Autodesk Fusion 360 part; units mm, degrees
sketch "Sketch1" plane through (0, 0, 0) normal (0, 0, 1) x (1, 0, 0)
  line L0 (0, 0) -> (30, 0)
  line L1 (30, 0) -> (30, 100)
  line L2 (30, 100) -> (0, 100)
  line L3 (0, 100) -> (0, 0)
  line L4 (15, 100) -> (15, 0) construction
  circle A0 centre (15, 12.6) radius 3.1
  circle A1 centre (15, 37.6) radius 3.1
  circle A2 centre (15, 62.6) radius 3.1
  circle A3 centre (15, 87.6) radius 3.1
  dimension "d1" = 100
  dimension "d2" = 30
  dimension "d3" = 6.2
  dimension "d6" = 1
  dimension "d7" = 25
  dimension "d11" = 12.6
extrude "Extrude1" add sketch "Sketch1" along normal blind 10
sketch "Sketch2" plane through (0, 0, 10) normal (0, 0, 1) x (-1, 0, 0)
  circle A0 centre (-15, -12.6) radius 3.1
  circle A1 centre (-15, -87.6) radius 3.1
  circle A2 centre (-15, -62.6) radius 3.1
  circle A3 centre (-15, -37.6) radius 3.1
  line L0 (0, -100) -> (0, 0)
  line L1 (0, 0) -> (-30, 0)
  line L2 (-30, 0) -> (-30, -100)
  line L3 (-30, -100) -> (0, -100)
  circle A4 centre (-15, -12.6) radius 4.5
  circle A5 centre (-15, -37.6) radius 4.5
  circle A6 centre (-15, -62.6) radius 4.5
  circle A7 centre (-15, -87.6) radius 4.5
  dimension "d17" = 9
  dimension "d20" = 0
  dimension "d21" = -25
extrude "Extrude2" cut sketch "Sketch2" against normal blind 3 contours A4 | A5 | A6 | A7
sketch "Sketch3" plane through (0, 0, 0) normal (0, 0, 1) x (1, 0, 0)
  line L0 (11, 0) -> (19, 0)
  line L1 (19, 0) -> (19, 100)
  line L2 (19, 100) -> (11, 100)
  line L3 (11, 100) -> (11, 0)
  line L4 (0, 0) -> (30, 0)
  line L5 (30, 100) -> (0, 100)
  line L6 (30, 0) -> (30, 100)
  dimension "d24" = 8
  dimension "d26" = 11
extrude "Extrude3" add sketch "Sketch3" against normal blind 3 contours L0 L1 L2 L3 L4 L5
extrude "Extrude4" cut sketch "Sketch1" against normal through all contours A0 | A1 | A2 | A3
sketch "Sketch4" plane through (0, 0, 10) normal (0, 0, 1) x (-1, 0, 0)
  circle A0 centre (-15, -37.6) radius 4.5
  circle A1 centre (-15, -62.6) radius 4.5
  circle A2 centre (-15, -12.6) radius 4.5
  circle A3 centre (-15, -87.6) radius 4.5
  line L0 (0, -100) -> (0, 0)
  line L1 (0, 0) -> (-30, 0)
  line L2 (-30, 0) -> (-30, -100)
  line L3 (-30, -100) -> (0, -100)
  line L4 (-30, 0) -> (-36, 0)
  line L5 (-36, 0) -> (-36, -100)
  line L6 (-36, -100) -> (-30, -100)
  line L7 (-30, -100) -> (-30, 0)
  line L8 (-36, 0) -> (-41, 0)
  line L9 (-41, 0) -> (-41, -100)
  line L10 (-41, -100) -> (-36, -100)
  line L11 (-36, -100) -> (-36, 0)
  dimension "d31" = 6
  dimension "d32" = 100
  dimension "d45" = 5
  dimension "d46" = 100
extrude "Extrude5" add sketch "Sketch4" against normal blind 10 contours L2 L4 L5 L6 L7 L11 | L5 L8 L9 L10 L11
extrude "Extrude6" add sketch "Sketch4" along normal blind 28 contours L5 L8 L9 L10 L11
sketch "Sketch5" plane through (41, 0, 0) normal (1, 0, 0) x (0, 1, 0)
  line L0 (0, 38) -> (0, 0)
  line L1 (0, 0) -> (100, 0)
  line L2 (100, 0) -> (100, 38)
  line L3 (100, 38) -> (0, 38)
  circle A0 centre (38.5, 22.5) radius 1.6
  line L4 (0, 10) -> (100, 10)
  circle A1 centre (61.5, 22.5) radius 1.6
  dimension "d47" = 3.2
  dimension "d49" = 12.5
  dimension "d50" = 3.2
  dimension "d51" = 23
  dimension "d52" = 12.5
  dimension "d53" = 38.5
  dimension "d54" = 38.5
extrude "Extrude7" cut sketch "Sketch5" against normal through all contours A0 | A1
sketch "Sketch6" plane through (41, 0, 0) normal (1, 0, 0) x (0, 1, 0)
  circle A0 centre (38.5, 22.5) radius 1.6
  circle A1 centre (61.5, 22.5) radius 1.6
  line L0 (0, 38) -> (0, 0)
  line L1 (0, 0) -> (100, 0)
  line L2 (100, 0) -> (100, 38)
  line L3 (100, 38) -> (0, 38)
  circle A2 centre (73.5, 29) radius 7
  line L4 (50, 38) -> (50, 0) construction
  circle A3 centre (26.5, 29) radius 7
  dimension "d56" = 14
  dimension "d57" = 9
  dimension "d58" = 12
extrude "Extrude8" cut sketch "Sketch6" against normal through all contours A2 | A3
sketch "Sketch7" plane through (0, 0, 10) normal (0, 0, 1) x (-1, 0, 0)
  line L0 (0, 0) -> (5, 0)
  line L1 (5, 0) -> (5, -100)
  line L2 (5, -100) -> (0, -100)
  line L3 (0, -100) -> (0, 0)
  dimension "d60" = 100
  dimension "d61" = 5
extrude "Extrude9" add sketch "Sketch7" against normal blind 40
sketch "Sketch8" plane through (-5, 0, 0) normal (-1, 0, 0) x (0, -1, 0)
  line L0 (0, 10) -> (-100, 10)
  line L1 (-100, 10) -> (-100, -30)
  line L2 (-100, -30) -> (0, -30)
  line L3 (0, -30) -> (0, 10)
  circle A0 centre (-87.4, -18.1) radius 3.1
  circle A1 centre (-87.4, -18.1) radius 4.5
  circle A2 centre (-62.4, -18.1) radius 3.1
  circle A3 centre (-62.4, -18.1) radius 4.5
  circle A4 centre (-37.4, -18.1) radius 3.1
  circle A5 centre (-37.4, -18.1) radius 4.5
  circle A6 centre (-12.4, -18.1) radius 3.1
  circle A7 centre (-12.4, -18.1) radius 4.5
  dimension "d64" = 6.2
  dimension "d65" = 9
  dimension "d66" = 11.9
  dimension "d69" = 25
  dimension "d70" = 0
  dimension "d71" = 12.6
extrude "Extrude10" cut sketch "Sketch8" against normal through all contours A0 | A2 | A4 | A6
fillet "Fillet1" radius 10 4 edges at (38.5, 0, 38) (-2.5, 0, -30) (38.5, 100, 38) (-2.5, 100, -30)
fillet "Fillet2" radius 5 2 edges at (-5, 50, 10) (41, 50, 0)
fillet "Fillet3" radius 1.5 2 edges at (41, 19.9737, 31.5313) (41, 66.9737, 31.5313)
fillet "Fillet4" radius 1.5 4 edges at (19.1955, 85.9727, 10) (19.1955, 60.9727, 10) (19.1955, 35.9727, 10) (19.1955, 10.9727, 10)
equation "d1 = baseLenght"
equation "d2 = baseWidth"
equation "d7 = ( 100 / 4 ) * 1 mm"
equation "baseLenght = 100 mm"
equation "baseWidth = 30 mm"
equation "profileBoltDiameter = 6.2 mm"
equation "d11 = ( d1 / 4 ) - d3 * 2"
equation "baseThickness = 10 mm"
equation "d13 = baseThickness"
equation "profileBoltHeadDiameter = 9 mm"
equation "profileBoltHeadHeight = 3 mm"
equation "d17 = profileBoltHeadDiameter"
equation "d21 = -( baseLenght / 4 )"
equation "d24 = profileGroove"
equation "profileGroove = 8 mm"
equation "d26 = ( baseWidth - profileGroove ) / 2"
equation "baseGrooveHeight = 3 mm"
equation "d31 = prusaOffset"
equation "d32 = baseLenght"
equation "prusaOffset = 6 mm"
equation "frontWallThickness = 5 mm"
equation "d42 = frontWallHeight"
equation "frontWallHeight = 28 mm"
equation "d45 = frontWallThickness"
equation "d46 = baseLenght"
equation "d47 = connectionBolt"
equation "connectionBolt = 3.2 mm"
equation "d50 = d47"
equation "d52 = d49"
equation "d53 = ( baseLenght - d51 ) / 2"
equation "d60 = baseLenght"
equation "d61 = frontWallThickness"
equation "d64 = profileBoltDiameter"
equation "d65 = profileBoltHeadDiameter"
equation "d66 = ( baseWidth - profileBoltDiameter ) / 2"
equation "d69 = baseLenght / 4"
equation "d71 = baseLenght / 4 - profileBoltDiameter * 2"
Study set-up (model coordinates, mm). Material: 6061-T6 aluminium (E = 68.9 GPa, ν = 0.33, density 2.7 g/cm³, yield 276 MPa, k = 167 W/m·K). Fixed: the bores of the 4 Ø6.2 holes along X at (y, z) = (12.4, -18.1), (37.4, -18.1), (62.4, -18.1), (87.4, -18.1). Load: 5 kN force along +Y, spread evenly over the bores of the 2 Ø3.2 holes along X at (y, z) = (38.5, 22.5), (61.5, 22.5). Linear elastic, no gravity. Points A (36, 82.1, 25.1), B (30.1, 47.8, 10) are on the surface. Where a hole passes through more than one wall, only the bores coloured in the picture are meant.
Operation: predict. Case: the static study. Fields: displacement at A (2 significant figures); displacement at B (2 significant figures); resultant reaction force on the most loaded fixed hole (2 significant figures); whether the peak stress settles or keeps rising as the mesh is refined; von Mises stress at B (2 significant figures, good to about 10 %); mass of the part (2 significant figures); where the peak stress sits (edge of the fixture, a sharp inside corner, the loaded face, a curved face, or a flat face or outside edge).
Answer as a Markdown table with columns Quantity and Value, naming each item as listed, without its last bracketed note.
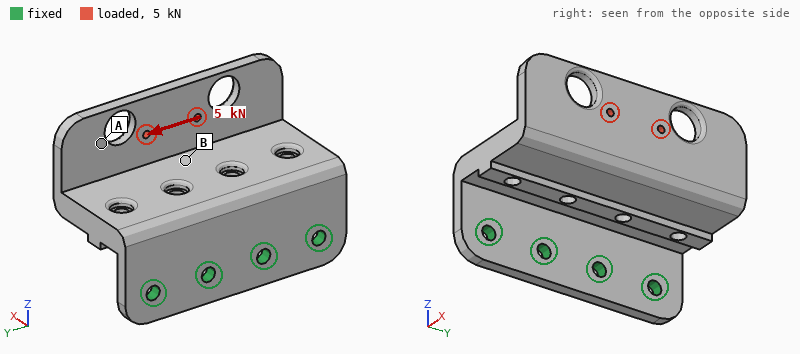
| Quantity | Value |
|---|---|
| displacement at A | 0.17 mm |
| displacement at B | 0.11 mm |
| resultant reaction force on the most loaded fixed hole | 3.5 kN |
| whether the peak stress settles or keeps rising as the mesh is refined | keeps rising |
| von Mises stress at B | 40 MPa |
| mass of the part | 190 g |
| where the peak stress sits | edge of the fixture |
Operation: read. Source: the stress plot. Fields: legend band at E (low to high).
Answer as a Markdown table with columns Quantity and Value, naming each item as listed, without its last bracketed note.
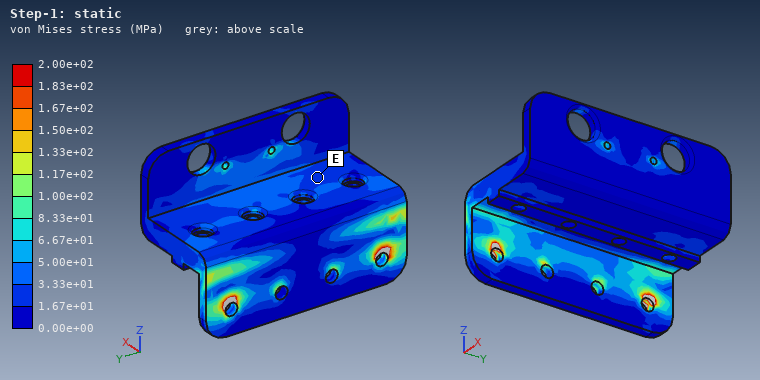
| Quantity | Value |
|---|---|
| legend band at E | 1.67e+01 to 3.33e+01 MPa |
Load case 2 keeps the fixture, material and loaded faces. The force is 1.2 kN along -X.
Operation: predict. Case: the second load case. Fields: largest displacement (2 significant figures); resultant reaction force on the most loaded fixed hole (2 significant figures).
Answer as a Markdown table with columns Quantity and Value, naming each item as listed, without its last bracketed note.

| Quantity | Value |
|---|---|
| largest displacement | 0.70 mm |
| resultant reaction force on the most loaded fixed hole | 330 N |
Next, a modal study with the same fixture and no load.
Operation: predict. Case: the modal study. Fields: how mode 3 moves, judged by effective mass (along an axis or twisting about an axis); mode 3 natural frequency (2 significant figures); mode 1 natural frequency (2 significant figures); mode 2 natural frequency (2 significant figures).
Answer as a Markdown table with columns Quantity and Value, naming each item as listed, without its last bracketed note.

| Quantity | Value |
|---|---|
| how mode 3 moves, judged by effective mass | along Y |
| mode 3 natural frequency | 3000 Hz |
| mode 1 natural frequency | 720 Hz |
| mode 2 natural frequency | 2100 Hz |
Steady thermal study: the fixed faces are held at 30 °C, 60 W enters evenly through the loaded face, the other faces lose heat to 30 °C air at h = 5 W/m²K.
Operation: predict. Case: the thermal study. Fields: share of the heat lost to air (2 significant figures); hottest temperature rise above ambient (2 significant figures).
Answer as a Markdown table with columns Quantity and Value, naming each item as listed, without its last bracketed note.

| Quantity | Value |
|---|---|
| share of the heat lost to air | 4.3 % |
| hottest temperature rise above ambient | 57 K |
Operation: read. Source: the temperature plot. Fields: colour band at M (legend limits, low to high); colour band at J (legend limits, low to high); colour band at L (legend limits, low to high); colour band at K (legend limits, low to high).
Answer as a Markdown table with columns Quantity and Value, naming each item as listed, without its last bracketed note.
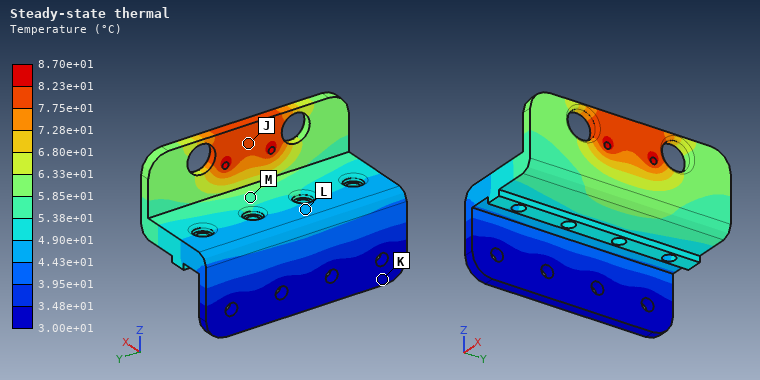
| Quantity | Value |
|---|---|
| colour band at M | 5.38e+01 to 5.85e+01 °C |
| colour band at J | 7.75e+01 to 8.23e+01 °C |
| colour band at L | 4.43e+01 to 4.90e+01 °C |
| colour band at K | 3.00e+01 to 3.48e+01 °C |
